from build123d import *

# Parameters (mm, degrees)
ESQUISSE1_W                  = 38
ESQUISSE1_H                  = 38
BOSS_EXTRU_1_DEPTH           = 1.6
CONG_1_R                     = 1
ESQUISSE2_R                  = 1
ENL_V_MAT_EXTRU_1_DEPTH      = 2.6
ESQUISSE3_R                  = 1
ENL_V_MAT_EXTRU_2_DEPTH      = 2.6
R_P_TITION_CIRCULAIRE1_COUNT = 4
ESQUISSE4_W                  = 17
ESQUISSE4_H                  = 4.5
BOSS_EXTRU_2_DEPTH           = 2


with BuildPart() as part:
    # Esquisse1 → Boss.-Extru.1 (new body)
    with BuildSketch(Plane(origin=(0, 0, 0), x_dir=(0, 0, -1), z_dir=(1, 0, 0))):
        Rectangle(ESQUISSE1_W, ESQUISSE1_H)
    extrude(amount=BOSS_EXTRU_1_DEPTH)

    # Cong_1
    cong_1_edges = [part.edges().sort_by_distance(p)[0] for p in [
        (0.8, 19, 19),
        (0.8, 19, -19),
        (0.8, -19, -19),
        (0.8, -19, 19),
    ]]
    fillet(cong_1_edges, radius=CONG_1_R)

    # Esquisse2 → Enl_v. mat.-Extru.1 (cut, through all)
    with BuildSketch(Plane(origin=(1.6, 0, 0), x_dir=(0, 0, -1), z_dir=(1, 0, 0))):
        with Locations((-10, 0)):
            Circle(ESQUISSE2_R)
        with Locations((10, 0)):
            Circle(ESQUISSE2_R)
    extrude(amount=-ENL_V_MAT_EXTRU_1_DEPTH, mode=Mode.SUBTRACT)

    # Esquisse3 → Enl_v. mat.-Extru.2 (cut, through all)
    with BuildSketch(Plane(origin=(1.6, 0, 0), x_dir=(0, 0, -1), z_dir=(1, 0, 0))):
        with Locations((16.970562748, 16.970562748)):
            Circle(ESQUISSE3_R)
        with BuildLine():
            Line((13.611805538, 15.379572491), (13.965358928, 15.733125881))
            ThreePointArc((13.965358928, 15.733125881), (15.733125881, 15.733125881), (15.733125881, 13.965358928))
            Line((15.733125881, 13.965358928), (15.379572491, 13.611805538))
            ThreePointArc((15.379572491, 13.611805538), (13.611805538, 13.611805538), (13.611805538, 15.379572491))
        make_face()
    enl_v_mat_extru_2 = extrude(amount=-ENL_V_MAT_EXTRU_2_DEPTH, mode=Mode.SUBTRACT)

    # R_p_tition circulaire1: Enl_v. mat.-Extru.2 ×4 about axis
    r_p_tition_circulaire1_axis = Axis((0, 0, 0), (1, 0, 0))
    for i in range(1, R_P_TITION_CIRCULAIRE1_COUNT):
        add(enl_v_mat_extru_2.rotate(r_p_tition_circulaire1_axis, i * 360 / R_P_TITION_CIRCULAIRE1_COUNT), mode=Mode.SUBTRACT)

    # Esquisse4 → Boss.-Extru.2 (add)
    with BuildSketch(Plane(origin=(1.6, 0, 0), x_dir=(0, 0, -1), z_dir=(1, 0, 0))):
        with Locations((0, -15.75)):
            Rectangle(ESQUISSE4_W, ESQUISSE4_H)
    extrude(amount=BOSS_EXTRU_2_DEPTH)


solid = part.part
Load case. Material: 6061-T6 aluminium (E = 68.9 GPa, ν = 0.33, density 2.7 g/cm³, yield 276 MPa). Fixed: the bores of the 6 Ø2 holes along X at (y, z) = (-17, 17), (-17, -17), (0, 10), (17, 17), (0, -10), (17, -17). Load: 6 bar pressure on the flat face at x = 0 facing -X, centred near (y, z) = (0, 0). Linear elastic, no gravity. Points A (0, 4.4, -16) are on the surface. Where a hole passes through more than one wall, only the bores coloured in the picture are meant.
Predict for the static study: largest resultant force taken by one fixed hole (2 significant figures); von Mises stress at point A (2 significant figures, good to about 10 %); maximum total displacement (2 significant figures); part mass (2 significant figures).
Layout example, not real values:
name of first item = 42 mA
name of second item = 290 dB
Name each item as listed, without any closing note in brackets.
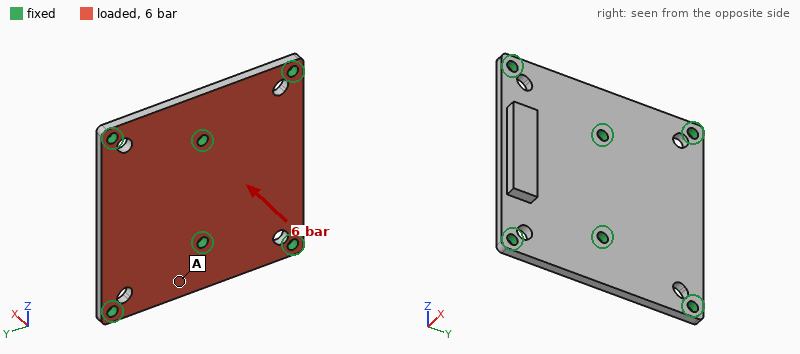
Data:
largest resultant force taken by one fixed hole = 230 N
von Mises stress at point A = 22 MPa
maximum total displacement = 84 µm
part mass = 6.5 g
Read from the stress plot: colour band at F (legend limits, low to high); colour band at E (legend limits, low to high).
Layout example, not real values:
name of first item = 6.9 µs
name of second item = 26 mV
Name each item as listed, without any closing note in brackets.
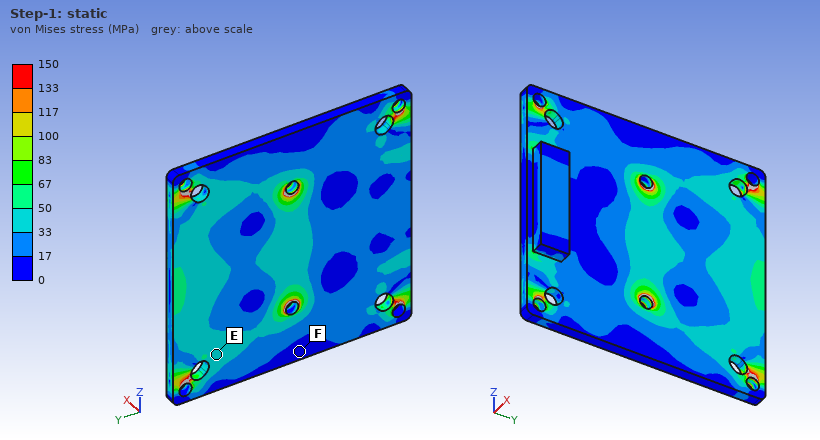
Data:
colour band at F = 0 to 17 MPa
colour band at E = 33 to 50 MPa
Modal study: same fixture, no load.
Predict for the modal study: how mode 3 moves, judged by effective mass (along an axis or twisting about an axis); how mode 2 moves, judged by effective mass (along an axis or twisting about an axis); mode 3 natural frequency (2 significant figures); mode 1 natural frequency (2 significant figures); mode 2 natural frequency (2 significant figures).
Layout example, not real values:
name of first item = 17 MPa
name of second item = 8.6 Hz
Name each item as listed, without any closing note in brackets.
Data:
how mode 3 moves, judged by effective mass = along X
how mode 2 moves, judged by effective mass = along X
mode 3 natural frequency = 18 kHz
mode 1 natural frequency = 8400 Hz
mode 2 natural frequency = 9200 Hz
